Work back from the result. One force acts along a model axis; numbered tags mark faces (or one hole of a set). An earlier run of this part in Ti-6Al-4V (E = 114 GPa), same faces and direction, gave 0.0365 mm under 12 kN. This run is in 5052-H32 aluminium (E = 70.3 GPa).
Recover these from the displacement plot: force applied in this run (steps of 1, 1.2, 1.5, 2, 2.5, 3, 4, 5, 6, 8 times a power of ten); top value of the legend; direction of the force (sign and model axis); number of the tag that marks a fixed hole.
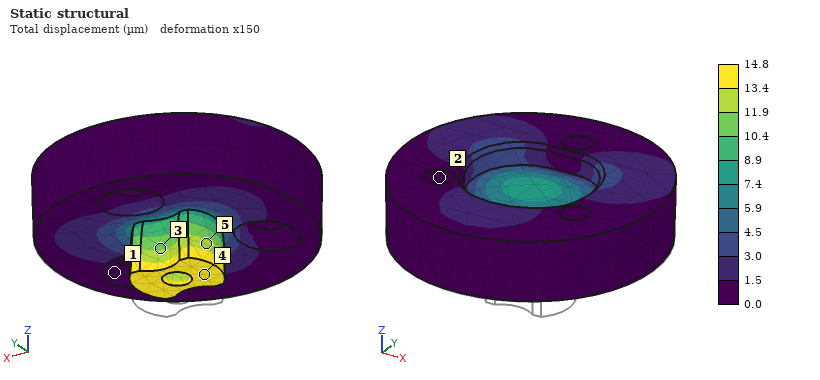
3 kN
14.8 µm
+Z
2
